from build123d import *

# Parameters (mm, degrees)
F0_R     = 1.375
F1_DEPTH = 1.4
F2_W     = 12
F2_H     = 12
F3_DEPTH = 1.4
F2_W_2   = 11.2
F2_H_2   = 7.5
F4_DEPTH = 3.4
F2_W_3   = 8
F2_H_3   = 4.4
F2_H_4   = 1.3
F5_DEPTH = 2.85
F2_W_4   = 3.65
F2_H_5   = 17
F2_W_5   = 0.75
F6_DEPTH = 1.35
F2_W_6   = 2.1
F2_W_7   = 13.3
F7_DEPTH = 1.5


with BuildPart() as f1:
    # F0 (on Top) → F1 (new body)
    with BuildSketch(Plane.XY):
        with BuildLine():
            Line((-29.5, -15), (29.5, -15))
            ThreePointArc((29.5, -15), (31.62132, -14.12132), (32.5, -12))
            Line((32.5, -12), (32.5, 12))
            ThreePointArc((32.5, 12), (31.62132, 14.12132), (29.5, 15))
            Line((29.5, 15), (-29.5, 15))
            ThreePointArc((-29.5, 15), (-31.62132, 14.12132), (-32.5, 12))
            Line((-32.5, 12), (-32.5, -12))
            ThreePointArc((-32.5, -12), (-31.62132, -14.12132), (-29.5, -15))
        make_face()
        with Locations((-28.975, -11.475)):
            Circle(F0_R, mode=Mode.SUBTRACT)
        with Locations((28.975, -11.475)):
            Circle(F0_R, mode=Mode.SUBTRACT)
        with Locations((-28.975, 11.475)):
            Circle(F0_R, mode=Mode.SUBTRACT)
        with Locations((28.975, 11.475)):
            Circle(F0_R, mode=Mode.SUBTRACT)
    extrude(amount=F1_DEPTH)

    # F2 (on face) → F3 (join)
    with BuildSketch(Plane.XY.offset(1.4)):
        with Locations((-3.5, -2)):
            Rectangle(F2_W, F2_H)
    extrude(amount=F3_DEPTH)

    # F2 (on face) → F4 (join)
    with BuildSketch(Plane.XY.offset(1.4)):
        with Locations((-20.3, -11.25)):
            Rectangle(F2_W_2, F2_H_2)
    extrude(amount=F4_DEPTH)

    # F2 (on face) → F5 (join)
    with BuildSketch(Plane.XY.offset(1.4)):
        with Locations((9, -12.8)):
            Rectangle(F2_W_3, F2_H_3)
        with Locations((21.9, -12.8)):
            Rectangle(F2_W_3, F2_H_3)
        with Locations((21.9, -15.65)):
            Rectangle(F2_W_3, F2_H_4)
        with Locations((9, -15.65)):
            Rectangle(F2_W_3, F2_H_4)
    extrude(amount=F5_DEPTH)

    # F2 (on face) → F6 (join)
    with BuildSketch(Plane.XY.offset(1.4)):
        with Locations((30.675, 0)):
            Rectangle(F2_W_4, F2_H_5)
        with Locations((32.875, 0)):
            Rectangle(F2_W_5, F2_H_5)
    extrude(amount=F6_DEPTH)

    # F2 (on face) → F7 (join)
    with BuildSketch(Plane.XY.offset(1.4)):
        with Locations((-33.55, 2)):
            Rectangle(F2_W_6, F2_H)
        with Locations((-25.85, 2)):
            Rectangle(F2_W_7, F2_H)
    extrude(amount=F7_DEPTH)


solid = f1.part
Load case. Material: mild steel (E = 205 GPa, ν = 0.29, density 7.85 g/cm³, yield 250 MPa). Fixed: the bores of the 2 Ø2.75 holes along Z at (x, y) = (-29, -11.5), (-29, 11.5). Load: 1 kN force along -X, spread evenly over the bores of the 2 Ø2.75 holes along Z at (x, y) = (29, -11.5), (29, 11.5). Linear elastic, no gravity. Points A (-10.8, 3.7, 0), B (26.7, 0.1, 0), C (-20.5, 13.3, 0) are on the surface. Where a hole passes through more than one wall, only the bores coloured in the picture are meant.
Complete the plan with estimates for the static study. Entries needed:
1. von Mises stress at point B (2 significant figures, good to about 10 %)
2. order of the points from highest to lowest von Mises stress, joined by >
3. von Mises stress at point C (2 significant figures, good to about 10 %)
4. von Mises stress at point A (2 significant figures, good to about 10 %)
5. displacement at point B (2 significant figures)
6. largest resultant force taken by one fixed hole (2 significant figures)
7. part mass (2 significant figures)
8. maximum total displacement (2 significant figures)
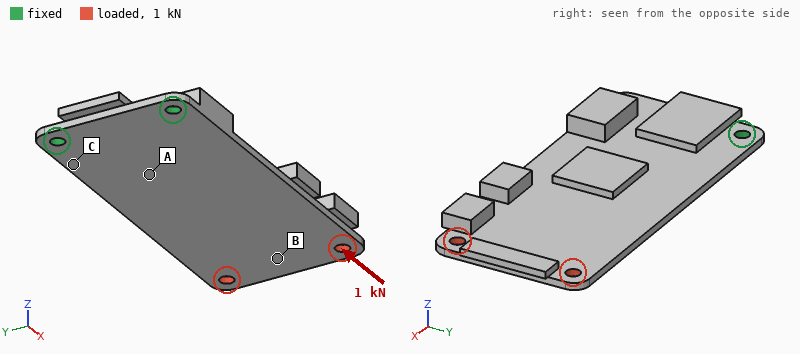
9.5 MPa
C > A > B
37 MPa
23 MPa
40 µm
510 N
30 g
49 µm
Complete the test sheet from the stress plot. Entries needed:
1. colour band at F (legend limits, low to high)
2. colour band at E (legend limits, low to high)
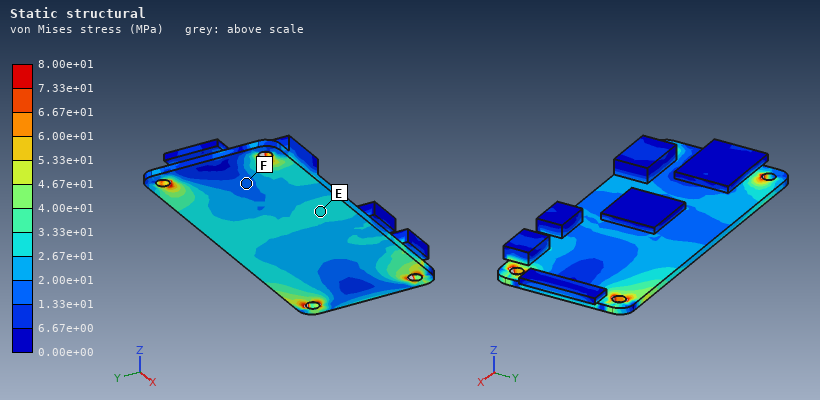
1.33e+01 to 2.00e+01 MPa
2.67e+01 to 3.33e+01 MPa
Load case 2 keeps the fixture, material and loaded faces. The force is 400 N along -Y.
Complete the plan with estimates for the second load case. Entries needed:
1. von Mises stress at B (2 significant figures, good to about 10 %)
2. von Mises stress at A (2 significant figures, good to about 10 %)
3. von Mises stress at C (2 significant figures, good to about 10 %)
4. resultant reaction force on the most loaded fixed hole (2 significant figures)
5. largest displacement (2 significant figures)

18 MPa
31 MPa
80 MPa
1.0 kN
66 µm
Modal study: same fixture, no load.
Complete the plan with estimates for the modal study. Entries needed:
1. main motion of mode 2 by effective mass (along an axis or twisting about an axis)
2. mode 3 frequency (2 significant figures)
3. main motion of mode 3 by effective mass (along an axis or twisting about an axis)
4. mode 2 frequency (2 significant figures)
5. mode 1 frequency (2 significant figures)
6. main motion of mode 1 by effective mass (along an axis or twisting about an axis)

twisting about X
2000 Hz
along Z
1600 Hz
360 Hz
along Z
